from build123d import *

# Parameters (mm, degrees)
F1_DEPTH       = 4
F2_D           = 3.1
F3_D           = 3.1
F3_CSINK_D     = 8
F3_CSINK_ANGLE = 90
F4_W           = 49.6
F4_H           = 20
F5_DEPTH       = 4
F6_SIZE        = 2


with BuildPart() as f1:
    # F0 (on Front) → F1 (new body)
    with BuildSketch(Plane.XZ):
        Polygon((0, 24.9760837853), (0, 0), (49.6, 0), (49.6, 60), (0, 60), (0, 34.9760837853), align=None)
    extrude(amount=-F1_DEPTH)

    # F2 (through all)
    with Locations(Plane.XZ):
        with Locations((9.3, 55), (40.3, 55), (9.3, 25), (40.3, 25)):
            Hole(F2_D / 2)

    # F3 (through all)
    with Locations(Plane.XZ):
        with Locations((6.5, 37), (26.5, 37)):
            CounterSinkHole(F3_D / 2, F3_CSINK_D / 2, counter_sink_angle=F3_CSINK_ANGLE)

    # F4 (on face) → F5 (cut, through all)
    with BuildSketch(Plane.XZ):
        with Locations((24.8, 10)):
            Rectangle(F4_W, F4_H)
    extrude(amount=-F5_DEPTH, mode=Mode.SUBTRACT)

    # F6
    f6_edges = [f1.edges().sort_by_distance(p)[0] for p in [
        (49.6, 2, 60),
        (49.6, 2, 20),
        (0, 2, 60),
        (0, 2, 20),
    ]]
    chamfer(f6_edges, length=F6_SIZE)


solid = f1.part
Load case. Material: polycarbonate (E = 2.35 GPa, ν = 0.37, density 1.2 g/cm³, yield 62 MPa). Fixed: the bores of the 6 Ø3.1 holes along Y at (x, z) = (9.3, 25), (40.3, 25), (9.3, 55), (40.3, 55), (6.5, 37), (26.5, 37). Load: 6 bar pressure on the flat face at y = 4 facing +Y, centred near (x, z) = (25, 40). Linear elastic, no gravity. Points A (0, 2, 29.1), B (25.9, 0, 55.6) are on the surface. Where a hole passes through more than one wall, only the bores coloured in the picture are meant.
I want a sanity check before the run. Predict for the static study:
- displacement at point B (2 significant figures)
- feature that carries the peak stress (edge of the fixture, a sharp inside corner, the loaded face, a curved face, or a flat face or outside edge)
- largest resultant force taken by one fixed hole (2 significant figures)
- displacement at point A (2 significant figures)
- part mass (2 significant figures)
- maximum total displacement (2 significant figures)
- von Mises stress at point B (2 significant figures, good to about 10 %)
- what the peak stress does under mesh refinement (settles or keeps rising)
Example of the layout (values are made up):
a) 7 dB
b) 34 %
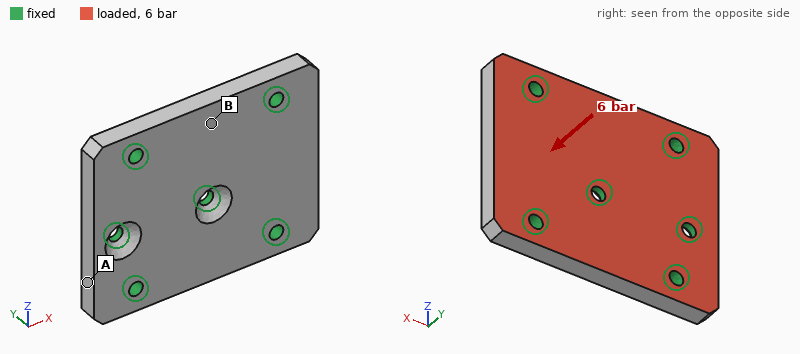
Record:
a) 0.11 mm
b) edge of the fixture
c) 240 N
d) 0.028 mm
e) 9.2 g
f) 0.18 mm
g) 6.5 MPa
h) keeps rising
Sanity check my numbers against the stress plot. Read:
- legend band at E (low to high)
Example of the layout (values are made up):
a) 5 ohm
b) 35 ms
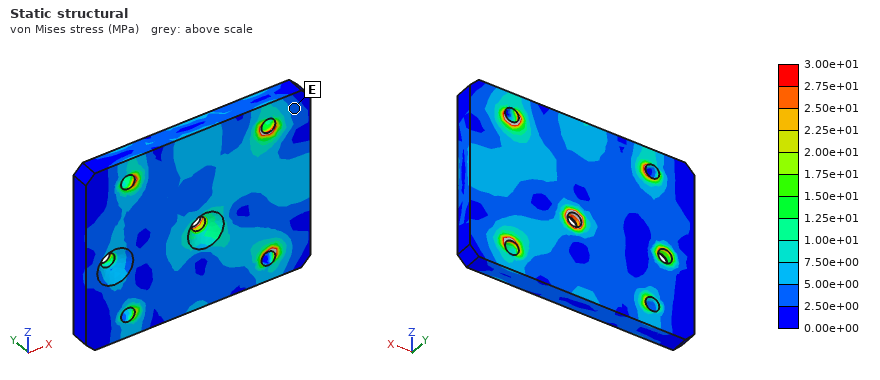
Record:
a) 2.50e+00 to 5.00e+00 MPa
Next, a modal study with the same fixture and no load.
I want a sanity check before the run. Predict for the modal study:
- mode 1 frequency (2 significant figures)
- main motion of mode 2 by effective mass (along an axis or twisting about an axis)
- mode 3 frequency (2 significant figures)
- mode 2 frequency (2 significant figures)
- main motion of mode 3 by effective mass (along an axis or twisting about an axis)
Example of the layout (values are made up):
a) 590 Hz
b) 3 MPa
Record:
a) 5300 Hz
b) along Y
c) 6800 Hz
d) 6100 Hz
e) along Y
